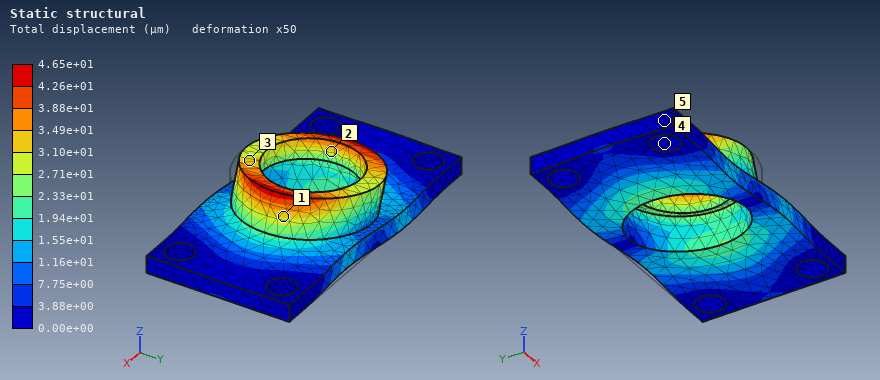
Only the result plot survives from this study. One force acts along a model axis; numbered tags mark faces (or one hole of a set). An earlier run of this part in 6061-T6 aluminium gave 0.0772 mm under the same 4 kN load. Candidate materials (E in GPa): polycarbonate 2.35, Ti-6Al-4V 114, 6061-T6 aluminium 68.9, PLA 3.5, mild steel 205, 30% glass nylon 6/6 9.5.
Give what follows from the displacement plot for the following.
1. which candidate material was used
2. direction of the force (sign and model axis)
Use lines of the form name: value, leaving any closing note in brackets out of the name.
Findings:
which candidate material was used: Ti-6Al-4V
direction of the force: -X
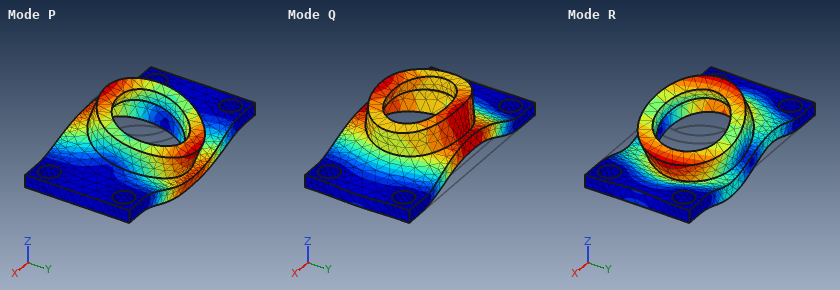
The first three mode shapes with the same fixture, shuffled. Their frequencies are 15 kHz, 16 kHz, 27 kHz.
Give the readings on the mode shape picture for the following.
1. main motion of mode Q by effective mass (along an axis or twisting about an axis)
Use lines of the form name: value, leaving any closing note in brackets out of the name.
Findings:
main motion of mode Q by effective mass: along Z
